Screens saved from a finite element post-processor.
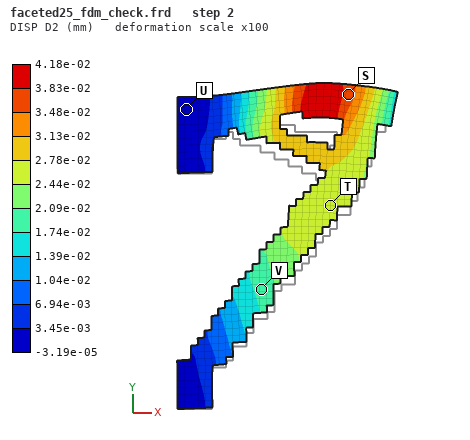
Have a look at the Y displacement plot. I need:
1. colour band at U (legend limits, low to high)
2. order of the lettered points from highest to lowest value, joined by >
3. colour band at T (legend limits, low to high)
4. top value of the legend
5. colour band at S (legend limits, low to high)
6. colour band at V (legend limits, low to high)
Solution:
-3.19e-05 to 3.45e-03 mm
S > T > V > U
2.44e-02 to 2.78e-02 mm
4.18e-02 mm
3.48e-02 to 3.83e-02 mm
1.74e-02 to 2.09e-02 mm
